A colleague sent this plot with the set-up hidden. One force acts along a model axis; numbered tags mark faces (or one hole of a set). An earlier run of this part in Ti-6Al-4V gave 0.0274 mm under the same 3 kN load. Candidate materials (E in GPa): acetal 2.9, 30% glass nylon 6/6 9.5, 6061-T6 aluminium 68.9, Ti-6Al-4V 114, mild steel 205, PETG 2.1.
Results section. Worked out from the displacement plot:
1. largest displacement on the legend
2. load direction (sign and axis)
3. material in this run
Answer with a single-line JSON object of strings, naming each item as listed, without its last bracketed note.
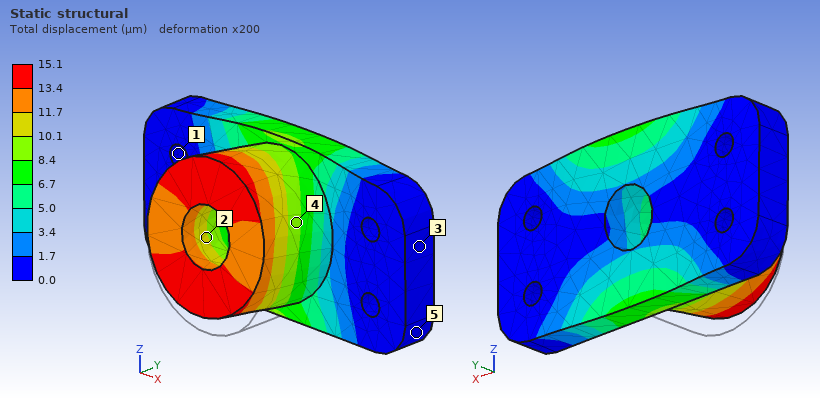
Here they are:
{"largest displacement on the legend": "15.1 µm", "load direction": "+Z", "material in this run": "mild steel"}
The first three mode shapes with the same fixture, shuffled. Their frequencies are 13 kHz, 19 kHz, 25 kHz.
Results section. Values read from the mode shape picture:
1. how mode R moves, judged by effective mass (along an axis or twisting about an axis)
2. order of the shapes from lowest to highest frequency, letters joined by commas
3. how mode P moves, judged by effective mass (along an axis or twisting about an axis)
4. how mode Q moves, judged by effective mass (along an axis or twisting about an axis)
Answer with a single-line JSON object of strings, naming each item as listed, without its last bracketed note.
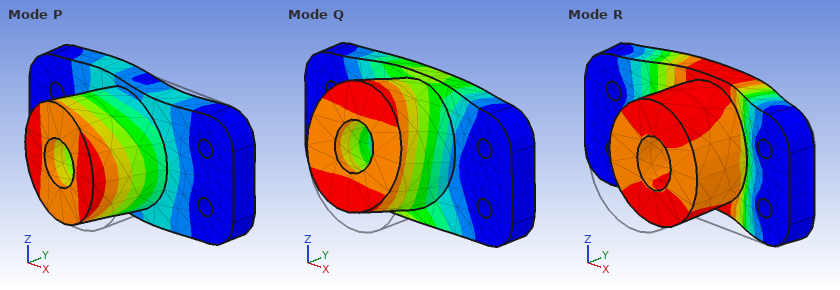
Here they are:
{"how mode R moves, judged by effective mass": "along Y", "order of the shapes from lowest to highest frequency, letters joined by commas": "Q, R, P", "how mode P moves, judged by effective mass": "along X", "how mode Q moves, judged by effective mass": "along Z"}
